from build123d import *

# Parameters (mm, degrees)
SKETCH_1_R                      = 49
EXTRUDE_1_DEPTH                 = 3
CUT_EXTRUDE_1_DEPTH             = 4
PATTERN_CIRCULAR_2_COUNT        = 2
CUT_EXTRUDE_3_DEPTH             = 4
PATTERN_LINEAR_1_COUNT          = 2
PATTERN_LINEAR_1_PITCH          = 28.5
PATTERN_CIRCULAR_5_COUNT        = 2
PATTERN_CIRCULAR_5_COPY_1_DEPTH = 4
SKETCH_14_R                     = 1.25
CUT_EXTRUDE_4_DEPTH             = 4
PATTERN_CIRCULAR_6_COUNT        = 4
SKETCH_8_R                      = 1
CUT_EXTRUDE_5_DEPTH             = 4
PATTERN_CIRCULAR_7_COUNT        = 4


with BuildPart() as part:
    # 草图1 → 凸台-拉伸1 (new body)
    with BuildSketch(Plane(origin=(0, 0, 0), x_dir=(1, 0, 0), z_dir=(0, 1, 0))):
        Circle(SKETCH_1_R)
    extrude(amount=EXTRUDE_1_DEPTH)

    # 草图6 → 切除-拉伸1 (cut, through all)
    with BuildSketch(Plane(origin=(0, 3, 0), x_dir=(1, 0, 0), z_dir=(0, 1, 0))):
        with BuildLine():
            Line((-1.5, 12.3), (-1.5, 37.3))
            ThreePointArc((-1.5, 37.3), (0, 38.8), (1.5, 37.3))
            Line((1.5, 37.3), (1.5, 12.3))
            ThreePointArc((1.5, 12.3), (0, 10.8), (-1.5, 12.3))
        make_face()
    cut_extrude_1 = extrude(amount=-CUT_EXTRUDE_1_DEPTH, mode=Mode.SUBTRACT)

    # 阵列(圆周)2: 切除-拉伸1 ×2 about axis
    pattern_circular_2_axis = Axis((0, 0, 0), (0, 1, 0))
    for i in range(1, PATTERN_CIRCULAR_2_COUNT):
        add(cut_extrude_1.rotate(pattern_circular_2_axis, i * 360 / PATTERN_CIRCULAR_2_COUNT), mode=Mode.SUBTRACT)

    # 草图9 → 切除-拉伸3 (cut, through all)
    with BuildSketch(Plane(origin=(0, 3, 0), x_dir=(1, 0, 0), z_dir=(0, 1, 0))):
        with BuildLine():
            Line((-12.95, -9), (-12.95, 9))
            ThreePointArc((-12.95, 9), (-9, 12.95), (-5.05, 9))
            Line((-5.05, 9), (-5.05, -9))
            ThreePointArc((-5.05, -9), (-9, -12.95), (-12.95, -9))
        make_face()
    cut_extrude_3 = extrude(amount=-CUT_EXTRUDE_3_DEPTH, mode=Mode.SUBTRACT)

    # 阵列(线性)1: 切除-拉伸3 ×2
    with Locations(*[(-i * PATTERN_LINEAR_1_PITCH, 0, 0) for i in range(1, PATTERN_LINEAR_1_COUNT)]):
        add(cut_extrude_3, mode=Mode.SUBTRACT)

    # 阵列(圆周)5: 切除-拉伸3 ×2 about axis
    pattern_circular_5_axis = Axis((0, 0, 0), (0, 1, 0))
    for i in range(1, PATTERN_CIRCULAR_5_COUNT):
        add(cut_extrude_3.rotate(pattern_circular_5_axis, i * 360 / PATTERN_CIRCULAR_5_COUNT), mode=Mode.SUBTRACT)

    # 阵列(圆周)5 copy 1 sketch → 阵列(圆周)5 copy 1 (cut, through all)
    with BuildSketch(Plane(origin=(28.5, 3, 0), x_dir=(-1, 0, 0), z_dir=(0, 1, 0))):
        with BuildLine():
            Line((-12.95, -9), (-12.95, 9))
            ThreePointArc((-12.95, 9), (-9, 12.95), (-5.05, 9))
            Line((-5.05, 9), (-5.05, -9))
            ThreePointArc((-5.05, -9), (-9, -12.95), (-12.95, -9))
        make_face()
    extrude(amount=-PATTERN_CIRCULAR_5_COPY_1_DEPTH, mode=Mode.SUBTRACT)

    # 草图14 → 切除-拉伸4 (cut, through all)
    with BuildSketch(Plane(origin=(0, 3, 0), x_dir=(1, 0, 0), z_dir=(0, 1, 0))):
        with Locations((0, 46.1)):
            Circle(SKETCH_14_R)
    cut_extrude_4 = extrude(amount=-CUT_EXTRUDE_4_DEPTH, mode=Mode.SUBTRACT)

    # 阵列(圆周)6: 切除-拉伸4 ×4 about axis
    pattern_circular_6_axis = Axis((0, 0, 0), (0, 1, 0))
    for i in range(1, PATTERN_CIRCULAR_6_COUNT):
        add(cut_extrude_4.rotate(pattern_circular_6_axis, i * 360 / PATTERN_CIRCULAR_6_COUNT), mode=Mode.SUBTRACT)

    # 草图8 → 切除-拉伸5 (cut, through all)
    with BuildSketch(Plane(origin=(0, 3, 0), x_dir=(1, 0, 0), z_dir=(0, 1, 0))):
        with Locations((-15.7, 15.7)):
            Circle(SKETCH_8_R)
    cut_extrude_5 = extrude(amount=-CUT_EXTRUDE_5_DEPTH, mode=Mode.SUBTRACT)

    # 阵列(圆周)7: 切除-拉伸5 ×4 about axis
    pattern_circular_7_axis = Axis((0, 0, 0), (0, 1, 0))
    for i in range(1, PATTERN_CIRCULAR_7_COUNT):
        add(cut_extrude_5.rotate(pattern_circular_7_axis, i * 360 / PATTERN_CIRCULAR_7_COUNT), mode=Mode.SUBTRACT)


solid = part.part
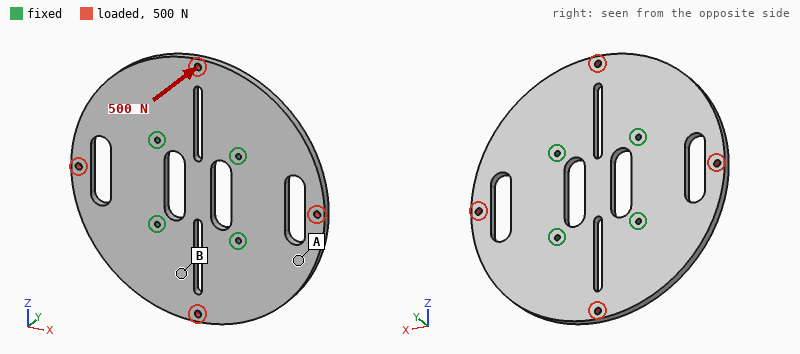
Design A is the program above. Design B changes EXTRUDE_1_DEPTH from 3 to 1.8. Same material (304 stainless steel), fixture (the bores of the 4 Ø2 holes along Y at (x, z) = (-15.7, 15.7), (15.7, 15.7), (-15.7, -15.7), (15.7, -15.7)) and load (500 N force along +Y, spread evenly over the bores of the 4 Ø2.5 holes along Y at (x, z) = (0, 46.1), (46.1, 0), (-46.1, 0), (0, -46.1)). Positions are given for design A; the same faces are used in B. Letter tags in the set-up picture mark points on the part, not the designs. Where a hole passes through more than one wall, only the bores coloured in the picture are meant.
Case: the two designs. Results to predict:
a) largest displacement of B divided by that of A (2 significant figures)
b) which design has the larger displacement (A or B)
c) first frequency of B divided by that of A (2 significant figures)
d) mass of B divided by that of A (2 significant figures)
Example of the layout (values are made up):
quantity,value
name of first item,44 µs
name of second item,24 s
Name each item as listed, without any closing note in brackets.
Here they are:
quantity,value
largest displacement of B divided by that of A,4.3
which design has the larger displacement,B
first frequency of B divided by that of A,0.63
mass of B divided by that of A,0.60
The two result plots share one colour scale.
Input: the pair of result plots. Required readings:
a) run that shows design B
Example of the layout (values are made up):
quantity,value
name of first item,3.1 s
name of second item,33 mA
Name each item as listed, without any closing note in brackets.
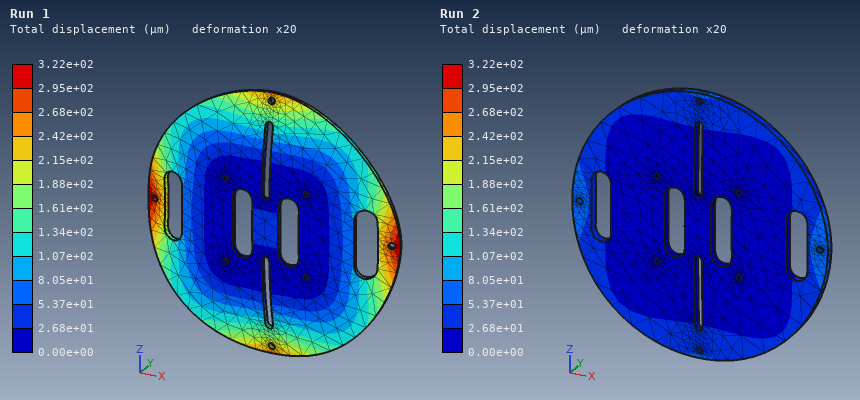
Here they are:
quantity,value
run that shows design B,Run 1
